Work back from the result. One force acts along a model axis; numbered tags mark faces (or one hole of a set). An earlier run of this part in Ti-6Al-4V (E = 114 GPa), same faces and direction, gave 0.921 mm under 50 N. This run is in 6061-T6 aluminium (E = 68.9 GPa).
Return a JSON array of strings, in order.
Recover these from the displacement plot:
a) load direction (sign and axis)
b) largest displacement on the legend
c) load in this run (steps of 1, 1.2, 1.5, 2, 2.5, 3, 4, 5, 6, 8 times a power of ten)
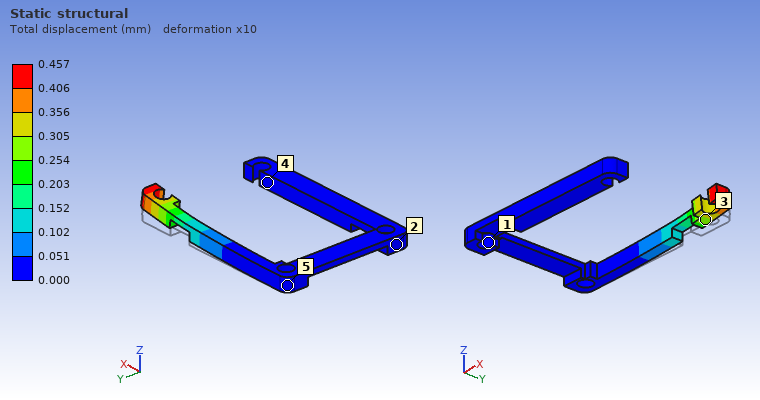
["+Z", "0.457 mm", "15 N"]
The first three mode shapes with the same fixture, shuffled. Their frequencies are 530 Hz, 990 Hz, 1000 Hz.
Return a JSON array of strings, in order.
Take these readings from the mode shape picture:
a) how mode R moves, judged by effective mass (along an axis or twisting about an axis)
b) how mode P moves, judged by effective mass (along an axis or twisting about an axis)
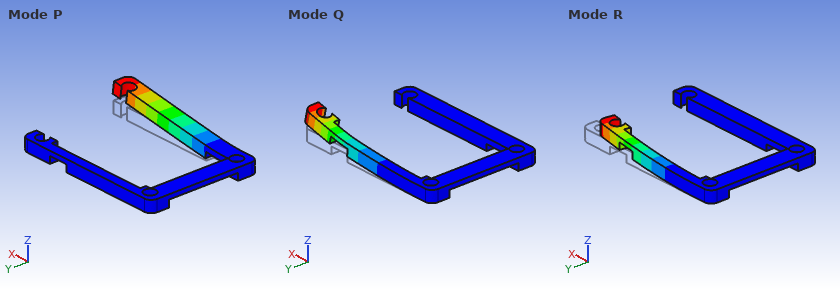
["along Y", "along Z"]
